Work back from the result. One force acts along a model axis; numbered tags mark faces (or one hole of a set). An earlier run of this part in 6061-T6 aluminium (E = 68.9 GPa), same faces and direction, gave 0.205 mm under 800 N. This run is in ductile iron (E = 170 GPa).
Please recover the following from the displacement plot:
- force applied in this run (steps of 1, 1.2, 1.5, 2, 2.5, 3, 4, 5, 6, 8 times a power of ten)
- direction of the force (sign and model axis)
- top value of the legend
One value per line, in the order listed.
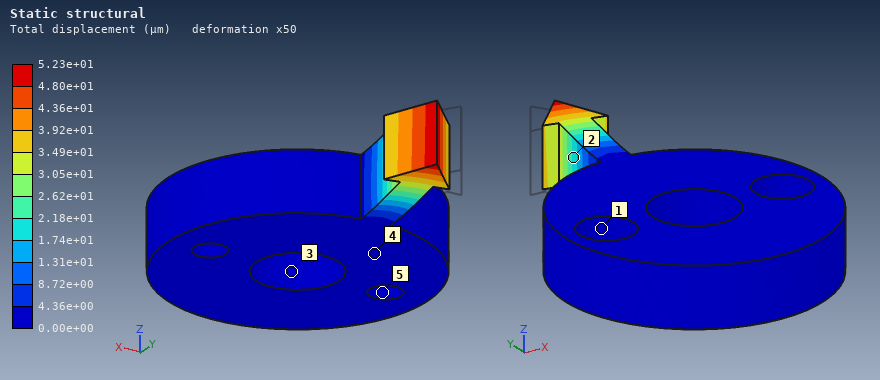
500 N
+X
5.23e+01 µm
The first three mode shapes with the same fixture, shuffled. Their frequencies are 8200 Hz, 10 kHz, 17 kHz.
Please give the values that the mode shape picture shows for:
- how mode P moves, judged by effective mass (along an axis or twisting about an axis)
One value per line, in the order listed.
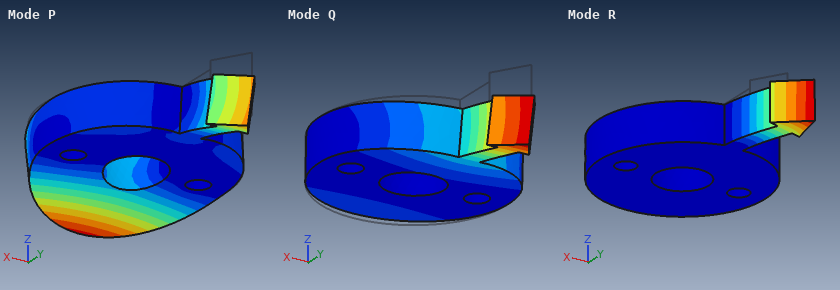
along Z
